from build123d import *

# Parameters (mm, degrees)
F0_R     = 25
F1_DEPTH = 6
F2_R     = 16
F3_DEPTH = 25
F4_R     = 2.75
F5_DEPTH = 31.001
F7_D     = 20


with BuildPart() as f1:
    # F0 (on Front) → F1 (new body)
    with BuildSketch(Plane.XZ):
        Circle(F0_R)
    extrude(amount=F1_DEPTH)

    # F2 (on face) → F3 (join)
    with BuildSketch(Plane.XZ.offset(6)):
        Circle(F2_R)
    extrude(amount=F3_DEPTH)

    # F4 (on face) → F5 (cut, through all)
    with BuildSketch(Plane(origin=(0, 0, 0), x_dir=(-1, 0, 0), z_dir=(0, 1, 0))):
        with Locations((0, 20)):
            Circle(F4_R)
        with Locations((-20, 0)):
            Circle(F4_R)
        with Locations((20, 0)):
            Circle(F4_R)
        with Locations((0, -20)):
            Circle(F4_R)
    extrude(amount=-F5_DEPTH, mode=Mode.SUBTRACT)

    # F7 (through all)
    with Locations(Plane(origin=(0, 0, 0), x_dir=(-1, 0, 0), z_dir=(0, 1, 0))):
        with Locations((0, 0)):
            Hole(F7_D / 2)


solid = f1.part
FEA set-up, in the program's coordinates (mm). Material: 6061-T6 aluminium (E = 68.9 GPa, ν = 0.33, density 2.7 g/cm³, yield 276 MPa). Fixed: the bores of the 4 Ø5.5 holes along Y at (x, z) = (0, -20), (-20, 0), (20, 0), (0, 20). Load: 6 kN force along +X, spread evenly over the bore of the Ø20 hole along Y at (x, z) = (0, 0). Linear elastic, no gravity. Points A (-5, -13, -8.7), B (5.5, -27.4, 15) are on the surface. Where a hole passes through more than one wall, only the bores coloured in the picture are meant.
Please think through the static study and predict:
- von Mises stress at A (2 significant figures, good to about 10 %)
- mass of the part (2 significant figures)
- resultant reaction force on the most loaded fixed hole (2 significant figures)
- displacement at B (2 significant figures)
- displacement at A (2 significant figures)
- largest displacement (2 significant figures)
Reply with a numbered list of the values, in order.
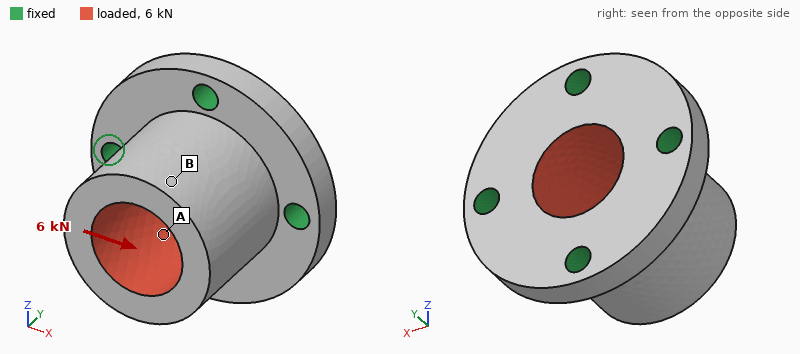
1. 23 MPa
2. 58 g
3. 2.6 kN
4. 20 µm
5. 9.7 µm
6. 25 µm
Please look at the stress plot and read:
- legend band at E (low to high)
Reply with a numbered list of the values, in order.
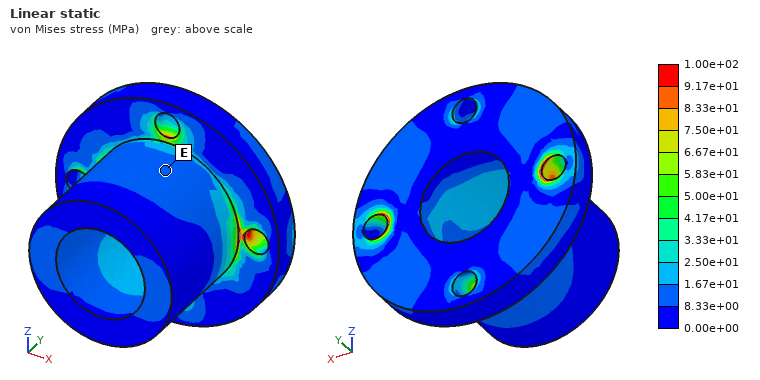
1. 8.33e+00 to 1.67e+01 MPa
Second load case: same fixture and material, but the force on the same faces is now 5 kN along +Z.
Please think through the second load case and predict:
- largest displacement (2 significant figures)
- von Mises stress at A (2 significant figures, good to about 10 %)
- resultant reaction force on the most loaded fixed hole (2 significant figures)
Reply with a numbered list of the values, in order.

1. 21 µm
2. 16 MPa
3. 2.2 kN
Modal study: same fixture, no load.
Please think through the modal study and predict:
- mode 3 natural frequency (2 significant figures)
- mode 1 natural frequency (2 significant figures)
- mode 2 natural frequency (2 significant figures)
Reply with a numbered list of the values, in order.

1. 23 kHz
2. 14 kHz
3. 14 kHz
